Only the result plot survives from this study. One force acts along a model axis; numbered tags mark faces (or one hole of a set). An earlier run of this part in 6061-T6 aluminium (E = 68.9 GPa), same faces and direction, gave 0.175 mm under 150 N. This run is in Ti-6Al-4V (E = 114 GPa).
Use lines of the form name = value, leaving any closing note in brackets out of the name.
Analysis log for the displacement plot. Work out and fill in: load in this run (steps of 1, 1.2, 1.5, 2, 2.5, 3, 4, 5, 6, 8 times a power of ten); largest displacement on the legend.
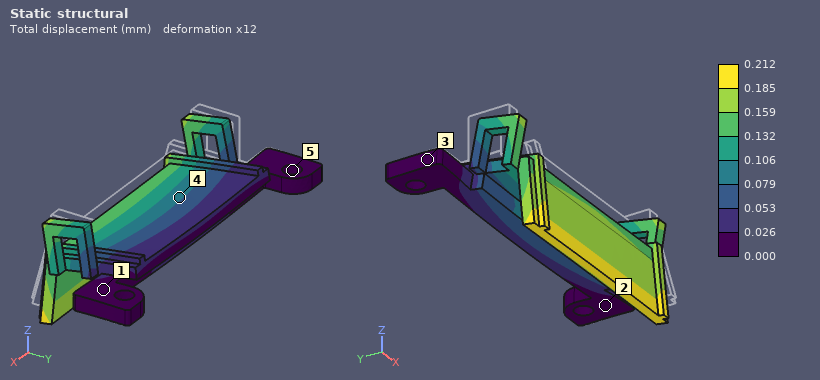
load in this run = 300 N
largest displacement on the legend = 0.212 mm
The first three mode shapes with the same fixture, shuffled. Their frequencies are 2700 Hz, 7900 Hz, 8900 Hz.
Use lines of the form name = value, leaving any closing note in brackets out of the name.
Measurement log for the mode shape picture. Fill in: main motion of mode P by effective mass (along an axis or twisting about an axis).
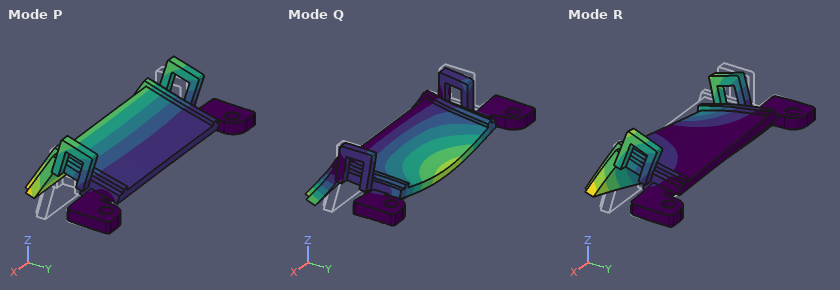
main motion of mode P by effective mass = along Z
